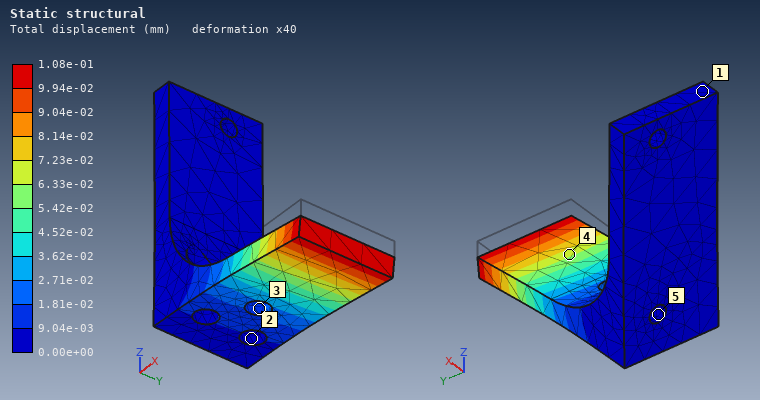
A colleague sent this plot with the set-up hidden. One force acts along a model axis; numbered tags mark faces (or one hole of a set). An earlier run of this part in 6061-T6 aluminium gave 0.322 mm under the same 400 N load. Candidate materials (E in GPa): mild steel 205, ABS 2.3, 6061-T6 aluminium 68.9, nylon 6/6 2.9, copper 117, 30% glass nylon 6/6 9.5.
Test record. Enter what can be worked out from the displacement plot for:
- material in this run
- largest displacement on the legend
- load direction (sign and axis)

mild steel
1.08e-01 mm
-Z
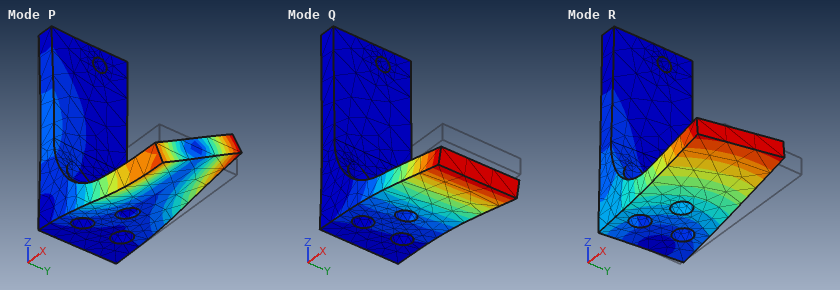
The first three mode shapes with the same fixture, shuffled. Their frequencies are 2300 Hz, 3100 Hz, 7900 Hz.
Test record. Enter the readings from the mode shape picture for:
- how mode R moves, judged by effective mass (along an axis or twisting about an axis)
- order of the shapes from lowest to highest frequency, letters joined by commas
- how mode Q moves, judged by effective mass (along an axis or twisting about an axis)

along Y
Q, R, P
along Z
